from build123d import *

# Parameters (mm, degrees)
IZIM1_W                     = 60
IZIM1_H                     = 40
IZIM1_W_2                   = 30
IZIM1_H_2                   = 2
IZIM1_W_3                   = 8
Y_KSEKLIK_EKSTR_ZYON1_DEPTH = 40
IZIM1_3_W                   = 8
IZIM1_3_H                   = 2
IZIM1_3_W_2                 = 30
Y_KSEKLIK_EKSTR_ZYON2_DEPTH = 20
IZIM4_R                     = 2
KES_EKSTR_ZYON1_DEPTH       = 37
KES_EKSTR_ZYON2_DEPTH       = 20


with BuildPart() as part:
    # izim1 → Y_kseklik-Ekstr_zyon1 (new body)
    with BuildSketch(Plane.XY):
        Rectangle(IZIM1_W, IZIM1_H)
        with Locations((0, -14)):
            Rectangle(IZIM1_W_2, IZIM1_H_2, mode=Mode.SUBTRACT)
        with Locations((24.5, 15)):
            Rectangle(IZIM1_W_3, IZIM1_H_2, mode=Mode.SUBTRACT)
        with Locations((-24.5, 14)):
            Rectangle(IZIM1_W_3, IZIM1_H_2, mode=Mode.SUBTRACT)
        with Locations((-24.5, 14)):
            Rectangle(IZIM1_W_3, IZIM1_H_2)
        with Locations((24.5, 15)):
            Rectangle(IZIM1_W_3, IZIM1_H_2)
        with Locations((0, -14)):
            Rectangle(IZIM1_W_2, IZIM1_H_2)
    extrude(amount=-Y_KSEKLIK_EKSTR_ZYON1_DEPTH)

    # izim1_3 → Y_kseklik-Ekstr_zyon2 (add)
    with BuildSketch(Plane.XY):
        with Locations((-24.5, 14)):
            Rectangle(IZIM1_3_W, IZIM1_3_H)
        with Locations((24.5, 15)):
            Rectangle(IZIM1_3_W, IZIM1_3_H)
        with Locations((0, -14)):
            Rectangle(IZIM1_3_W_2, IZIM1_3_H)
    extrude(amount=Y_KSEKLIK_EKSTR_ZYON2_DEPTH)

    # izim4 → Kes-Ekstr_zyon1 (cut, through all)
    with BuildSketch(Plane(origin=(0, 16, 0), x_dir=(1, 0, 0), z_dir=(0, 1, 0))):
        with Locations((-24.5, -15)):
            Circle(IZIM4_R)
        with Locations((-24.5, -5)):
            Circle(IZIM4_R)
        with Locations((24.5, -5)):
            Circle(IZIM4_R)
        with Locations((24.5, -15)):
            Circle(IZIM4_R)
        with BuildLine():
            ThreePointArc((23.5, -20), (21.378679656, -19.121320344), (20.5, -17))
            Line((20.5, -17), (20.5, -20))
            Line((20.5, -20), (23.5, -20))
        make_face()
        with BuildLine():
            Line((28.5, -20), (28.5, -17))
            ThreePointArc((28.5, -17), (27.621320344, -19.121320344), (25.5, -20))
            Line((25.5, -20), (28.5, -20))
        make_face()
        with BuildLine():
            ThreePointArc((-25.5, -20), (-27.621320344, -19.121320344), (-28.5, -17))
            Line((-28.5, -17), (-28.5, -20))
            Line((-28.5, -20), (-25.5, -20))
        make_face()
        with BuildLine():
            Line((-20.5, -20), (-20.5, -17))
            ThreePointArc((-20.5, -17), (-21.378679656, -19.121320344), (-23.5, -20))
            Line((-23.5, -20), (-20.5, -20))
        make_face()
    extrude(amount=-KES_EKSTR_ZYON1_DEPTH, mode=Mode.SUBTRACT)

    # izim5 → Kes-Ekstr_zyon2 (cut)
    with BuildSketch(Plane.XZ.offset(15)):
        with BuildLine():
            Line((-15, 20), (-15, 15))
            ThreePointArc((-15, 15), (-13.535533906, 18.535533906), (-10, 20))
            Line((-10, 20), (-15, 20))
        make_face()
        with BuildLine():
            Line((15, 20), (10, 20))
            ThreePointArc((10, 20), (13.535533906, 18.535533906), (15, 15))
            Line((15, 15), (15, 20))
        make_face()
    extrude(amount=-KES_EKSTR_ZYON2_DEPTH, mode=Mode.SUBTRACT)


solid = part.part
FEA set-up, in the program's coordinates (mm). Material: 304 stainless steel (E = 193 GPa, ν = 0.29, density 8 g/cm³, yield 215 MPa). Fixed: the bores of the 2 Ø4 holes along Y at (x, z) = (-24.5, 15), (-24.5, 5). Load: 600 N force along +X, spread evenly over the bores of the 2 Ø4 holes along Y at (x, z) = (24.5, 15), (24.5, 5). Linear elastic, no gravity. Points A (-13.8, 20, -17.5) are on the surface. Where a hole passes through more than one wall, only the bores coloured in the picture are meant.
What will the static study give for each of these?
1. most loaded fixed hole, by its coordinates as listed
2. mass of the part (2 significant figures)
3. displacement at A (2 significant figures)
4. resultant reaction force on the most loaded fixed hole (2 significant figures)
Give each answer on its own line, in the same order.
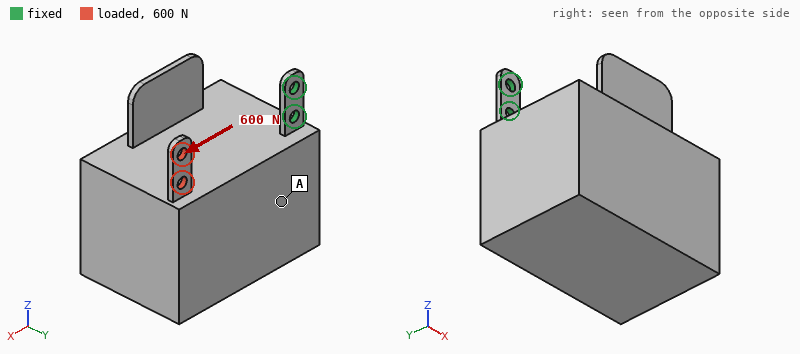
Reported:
(-24.5, 5)
780 g
0.038 mm
530 N
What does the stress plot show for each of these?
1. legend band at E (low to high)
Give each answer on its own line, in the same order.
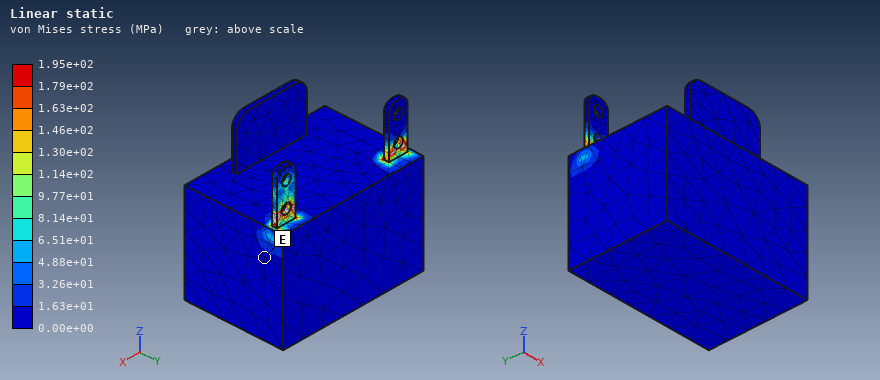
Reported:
0.00e+00 to 1.63e+01 MPa
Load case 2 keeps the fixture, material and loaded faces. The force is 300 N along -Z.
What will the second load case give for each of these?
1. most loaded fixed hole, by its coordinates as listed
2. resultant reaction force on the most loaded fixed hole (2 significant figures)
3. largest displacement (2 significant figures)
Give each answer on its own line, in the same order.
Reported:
(-24.5, 5)
400 N
0.42 mm
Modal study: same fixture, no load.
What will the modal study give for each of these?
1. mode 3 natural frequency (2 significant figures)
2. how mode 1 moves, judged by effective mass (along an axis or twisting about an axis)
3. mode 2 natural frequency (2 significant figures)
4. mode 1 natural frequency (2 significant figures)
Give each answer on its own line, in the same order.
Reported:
290 Hz
along Y
150 Hz
88 Hz
